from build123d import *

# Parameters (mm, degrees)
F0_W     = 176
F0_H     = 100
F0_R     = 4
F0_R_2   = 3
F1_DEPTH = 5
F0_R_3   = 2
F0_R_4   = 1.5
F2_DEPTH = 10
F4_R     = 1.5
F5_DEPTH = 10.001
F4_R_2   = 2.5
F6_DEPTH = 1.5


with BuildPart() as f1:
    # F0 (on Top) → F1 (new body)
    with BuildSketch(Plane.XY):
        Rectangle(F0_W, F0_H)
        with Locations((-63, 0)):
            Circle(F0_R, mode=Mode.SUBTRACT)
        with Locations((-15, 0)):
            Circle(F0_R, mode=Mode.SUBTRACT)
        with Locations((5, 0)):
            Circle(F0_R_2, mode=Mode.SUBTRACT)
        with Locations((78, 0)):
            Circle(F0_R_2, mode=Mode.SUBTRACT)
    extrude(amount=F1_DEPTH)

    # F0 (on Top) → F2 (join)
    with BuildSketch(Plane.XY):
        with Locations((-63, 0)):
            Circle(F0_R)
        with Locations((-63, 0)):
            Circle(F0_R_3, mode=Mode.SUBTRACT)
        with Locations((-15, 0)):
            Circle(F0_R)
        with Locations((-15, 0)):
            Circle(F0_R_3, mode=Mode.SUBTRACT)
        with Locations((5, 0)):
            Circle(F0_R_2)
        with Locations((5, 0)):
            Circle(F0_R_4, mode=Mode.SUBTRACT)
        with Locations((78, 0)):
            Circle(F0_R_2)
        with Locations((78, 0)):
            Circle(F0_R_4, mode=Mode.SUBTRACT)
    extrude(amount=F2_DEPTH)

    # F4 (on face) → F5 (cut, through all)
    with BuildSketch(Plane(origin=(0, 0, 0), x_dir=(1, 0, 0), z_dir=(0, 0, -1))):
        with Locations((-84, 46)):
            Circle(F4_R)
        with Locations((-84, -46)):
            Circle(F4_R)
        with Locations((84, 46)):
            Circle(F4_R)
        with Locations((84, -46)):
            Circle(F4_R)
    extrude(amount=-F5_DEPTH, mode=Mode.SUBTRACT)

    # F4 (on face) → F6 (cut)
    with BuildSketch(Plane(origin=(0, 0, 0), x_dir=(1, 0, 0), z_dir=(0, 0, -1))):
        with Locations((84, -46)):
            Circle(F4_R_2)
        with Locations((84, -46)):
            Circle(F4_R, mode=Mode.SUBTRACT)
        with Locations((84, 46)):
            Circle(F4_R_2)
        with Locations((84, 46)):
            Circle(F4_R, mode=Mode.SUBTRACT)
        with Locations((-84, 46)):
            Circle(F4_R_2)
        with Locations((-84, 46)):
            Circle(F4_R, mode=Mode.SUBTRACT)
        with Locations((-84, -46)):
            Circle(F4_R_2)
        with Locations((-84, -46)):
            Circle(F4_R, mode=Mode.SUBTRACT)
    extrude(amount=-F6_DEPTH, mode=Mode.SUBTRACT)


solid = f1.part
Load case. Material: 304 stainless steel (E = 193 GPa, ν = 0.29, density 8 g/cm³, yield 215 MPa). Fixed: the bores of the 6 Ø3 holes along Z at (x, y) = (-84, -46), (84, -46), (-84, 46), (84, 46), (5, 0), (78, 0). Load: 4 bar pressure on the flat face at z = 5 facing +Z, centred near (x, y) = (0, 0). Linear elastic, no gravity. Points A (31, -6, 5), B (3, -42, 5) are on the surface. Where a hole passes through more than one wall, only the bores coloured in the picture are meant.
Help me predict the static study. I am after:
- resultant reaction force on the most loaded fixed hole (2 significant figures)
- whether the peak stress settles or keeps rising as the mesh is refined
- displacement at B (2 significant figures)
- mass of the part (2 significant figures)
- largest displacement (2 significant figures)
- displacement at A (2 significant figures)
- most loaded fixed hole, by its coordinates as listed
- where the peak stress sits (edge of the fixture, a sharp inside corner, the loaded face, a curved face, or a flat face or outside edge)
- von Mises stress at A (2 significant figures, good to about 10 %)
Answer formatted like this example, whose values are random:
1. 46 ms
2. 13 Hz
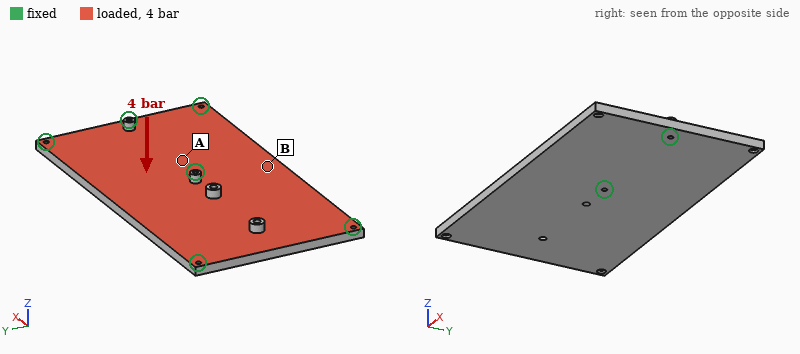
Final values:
1. 3.5 kN
2. keeps rising
3. 0.098 mm
4. 710 g
5. 0.13 mm
6. 0.023 mm
7. (5, 0)
8. edge of the fixture
9. 51 MPa
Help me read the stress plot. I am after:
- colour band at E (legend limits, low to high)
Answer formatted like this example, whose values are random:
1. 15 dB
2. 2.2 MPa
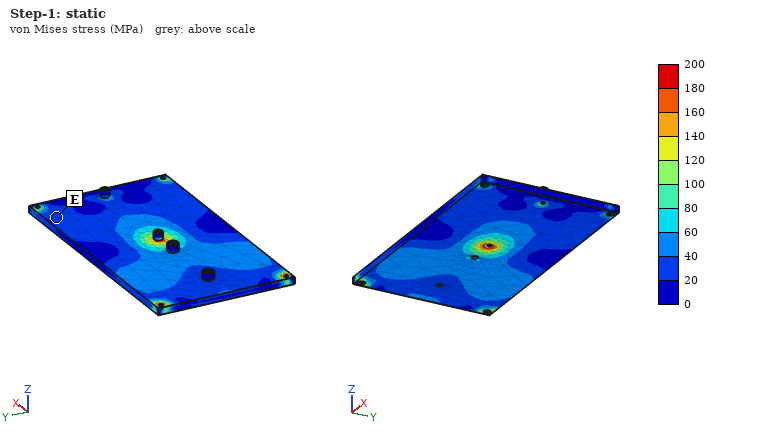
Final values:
1. 20 to 40 MPa
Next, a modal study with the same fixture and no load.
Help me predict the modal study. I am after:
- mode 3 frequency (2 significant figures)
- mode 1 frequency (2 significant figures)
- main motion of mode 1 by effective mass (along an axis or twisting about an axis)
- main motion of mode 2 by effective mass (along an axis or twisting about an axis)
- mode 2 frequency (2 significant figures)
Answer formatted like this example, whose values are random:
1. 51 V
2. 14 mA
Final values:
1. 2100 Hz
2. 1500 Hz
3. twisting about X
4. along Z
5. 1800 Hz
